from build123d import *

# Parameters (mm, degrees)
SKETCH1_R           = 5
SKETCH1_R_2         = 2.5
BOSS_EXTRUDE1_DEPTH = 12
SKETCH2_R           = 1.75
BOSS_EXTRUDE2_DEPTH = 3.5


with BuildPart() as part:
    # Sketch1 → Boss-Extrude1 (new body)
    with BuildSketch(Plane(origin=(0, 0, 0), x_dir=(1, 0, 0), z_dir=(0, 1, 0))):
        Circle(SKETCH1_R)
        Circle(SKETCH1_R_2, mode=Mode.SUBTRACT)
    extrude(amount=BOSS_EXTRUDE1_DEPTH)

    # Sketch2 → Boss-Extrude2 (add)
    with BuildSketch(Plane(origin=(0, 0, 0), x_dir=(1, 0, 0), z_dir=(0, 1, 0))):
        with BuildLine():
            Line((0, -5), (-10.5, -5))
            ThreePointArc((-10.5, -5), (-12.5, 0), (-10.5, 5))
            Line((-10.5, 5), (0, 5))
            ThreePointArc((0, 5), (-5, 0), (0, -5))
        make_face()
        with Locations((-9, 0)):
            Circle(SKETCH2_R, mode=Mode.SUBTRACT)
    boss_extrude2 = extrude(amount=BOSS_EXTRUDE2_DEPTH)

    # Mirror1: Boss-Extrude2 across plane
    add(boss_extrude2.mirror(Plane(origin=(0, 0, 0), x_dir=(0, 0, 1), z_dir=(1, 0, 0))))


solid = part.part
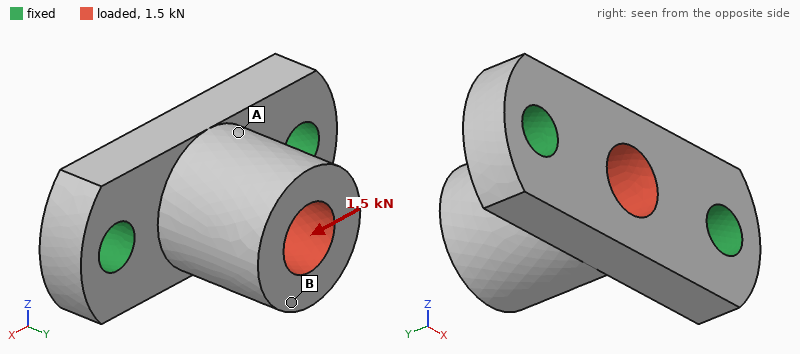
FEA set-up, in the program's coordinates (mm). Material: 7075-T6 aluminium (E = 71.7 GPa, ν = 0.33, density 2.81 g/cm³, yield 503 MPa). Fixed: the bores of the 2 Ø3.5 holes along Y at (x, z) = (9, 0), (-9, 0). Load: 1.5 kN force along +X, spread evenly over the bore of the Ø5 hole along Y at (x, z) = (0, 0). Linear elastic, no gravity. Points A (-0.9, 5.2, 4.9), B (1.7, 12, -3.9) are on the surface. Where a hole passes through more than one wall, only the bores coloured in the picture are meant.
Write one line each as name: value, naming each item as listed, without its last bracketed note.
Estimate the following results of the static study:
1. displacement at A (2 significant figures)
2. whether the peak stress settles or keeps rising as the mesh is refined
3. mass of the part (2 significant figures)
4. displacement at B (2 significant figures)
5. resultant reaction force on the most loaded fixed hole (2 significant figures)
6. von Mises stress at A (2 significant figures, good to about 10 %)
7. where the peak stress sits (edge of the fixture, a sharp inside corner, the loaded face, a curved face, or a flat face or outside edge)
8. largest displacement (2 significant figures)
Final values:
displacement at A: 5.5 µm
whether the peak stress settles or keeps rising as the mesh is refined: keeps rising
mass of the part: 3.4 g
displacement at B: 16 µm
resultant reaction force on the most loaded fixed hole: 890 N
von Mises stress at A: 24 MPa
where the peak stress sits: edge of the fixture
largest displacement: 17 µm
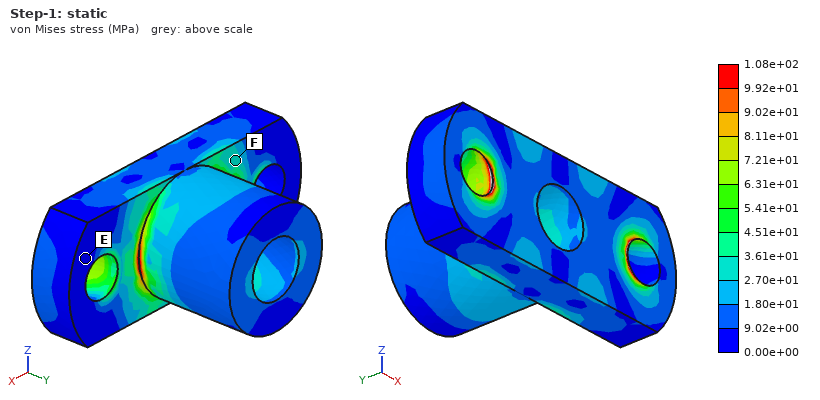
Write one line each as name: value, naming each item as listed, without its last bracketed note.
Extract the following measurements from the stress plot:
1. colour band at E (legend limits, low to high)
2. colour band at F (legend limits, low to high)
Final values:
colour band at E: 0.00e+00 to 9.02e+00 MPa
colour band at F: 2.70e+01 to 3.61e+01 MPa
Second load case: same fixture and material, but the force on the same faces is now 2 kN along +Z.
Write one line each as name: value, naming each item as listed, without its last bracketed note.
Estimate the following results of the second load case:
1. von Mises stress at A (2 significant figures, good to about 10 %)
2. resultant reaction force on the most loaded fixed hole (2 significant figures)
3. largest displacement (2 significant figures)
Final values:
von Mises stress at A: 35 MPa
resultant reaction force on the most loaded fixed hole: 1.0 kN
largest displacement: 84 µm
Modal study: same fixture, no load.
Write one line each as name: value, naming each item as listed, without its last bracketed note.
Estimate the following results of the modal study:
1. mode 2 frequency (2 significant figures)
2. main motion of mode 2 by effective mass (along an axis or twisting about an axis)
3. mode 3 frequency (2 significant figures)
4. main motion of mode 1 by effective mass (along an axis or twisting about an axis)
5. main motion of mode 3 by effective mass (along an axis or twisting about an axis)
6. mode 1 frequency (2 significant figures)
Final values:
mode 2 frequency: 39 kHz
main motion of mode 2 by effective mass: along X
mode 3 frequency: 42 kHz
main motion of mode 1 by effective mass: along Z
main motion of mode 3 by effective mass: along Y
mode 1 frequency: 20 kHz
